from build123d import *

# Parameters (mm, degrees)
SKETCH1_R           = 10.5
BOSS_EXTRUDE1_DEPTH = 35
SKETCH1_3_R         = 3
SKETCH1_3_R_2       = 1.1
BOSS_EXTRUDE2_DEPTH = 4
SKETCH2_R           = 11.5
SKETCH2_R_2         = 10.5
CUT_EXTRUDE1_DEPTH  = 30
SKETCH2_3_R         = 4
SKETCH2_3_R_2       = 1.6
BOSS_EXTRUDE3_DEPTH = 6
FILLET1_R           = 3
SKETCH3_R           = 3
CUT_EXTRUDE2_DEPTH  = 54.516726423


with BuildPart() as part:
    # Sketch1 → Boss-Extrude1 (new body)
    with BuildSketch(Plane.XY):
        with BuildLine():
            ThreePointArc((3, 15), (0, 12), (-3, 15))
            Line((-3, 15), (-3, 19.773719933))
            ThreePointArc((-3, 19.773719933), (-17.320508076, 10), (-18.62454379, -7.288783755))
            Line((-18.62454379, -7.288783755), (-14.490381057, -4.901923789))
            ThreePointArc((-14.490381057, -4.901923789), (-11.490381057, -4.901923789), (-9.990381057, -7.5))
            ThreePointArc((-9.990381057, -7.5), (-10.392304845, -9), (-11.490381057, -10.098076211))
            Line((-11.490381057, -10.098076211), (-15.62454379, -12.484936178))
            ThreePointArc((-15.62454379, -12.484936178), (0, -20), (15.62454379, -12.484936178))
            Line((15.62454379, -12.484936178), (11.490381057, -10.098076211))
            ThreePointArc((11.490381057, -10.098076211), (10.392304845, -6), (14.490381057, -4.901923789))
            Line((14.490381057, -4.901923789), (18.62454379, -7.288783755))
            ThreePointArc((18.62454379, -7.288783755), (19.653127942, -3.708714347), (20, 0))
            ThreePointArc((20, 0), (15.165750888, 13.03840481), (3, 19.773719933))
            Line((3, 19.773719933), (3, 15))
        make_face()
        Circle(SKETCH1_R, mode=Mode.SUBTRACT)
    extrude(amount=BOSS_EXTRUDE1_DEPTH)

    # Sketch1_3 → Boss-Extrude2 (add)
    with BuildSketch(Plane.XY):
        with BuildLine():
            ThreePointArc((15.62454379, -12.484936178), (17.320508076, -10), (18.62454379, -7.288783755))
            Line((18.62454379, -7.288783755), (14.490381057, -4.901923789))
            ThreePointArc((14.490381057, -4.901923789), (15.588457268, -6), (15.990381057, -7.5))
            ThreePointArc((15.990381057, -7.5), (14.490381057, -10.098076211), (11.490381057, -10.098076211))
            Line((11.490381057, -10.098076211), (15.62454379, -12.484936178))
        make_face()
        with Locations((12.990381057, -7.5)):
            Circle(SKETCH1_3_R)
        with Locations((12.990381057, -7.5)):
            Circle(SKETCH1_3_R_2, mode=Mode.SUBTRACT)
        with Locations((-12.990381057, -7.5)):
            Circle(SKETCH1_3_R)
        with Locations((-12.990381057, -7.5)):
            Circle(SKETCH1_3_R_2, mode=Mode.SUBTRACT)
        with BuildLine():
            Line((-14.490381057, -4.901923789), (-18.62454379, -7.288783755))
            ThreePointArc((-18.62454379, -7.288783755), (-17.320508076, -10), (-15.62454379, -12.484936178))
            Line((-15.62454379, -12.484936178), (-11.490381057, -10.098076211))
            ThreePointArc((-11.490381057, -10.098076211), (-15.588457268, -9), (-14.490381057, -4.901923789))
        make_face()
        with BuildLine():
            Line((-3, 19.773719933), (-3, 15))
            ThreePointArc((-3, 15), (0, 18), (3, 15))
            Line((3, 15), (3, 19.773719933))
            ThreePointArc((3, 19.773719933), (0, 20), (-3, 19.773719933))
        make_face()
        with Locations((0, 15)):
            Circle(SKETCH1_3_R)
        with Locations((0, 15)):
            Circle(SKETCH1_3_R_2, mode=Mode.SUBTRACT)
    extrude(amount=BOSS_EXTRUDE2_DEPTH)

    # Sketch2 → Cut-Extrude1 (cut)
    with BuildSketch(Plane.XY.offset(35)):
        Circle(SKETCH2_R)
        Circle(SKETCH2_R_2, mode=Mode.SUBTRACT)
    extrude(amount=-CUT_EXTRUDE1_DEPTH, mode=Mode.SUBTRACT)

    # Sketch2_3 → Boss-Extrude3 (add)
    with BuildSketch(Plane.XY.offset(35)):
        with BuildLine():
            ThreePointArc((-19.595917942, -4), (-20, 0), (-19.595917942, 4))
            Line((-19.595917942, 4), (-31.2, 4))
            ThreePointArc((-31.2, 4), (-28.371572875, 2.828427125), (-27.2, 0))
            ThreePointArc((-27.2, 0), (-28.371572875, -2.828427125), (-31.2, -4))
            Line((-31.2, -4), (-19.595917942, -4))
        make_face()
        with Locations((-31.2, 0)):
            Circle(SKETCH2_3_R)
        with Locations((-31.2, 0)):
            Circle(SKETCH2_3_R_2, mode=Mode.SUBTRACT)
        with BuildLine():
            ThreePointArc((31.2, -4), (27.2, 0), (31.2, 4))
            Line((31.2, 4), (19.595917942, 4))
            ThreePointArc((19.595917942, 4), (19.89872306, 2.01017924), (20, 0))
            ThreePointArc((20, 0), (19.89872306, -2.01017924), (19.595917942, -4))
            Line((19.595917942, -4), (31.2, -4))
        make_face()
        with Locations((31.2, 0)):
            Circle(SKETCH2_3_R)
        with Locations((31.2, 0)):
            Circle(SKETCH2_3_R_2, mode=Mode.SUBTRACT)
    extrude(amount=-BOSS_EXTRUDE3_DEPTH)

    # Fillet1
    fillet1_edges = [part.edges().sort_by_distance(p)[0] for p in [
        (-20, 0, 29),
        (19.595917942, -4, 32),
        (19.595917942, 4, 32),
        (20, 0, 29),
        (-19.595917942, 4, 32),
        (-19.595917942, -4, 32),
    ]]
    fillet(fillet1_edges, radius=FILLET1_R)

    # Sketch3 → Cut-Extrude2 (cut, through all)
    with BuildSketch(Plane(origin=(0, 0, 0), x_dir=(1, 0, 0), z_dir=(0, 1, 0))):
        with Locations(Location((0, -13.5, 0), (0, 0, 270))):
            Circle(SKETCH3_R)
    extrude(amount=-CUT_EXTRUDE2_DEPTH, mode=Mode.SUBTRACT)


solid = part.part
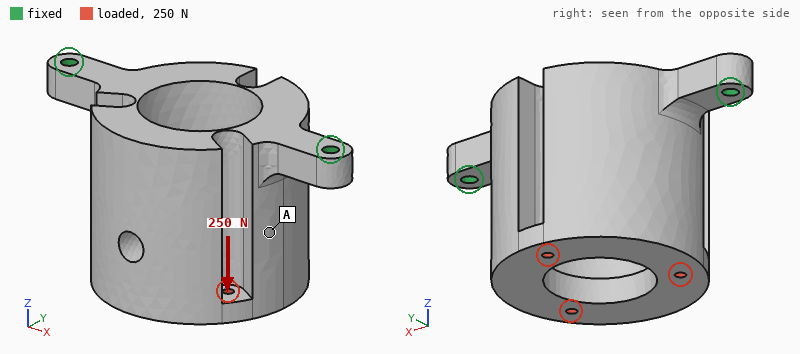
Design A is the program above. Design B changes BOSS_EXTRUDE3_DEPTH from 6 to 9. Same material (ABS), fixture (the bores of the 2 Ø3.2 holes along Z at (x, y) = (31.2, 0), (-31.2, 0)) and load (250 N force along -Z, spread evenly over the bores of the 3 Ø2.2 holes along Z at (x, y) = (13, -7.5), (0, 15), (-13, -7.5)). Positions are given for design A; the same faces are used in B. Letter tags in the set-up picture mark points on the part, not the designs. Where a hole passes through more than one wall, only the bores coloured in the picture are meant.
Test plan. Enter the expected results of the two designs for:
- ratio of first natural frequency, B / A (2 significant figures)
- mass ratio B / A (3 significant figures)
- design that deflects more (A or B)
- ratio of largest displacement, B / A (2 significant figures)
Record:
1.5
1.02
A
0.65
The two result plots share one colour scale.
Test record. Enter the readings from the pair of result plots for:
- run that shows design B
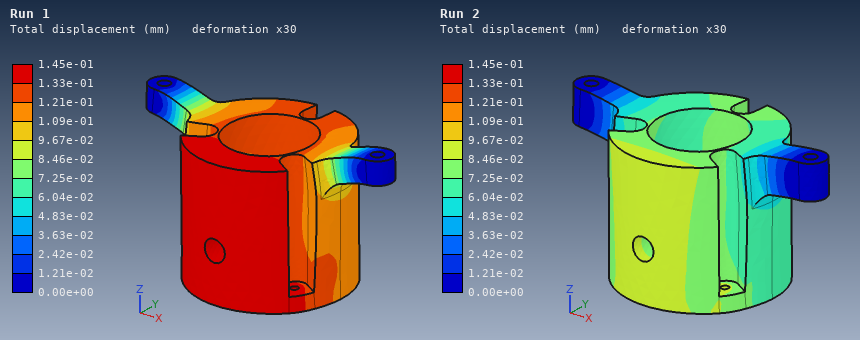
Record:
Run 2
